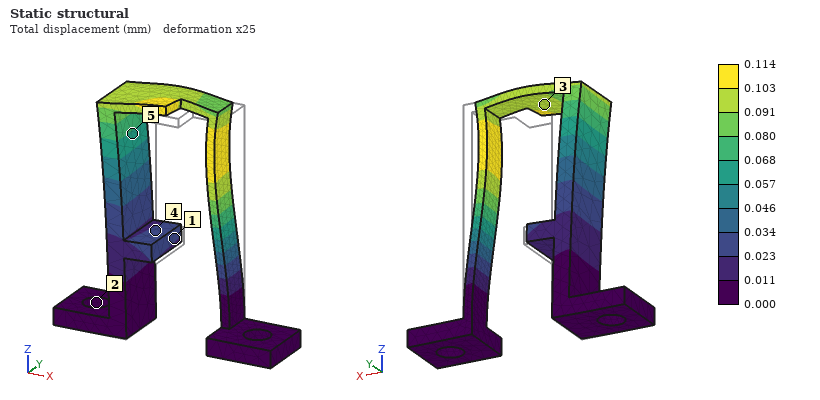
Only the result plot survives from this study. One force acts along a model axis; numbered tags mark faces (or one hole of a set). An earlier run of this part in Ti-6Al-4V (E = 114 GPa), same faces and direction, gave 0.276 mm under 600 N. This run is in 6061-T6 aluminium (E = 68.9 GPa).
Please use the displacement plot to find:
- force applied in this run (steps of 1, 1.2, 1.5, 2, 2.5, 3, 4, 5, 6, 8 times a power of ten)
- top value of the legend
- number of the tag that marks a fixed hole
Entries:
150 N
0.114 mm
2
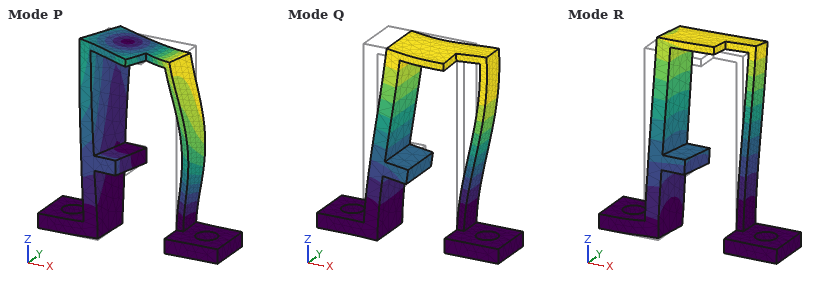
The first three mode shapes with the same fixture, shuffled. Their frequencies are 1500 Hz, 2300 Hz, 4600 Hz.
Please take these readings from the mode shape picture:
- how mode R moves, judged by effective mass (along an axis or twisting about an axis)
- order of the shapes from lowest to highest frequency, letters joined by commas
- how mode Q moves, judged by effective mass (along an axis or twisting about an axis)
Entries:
along Y
Q, R, P
along X
